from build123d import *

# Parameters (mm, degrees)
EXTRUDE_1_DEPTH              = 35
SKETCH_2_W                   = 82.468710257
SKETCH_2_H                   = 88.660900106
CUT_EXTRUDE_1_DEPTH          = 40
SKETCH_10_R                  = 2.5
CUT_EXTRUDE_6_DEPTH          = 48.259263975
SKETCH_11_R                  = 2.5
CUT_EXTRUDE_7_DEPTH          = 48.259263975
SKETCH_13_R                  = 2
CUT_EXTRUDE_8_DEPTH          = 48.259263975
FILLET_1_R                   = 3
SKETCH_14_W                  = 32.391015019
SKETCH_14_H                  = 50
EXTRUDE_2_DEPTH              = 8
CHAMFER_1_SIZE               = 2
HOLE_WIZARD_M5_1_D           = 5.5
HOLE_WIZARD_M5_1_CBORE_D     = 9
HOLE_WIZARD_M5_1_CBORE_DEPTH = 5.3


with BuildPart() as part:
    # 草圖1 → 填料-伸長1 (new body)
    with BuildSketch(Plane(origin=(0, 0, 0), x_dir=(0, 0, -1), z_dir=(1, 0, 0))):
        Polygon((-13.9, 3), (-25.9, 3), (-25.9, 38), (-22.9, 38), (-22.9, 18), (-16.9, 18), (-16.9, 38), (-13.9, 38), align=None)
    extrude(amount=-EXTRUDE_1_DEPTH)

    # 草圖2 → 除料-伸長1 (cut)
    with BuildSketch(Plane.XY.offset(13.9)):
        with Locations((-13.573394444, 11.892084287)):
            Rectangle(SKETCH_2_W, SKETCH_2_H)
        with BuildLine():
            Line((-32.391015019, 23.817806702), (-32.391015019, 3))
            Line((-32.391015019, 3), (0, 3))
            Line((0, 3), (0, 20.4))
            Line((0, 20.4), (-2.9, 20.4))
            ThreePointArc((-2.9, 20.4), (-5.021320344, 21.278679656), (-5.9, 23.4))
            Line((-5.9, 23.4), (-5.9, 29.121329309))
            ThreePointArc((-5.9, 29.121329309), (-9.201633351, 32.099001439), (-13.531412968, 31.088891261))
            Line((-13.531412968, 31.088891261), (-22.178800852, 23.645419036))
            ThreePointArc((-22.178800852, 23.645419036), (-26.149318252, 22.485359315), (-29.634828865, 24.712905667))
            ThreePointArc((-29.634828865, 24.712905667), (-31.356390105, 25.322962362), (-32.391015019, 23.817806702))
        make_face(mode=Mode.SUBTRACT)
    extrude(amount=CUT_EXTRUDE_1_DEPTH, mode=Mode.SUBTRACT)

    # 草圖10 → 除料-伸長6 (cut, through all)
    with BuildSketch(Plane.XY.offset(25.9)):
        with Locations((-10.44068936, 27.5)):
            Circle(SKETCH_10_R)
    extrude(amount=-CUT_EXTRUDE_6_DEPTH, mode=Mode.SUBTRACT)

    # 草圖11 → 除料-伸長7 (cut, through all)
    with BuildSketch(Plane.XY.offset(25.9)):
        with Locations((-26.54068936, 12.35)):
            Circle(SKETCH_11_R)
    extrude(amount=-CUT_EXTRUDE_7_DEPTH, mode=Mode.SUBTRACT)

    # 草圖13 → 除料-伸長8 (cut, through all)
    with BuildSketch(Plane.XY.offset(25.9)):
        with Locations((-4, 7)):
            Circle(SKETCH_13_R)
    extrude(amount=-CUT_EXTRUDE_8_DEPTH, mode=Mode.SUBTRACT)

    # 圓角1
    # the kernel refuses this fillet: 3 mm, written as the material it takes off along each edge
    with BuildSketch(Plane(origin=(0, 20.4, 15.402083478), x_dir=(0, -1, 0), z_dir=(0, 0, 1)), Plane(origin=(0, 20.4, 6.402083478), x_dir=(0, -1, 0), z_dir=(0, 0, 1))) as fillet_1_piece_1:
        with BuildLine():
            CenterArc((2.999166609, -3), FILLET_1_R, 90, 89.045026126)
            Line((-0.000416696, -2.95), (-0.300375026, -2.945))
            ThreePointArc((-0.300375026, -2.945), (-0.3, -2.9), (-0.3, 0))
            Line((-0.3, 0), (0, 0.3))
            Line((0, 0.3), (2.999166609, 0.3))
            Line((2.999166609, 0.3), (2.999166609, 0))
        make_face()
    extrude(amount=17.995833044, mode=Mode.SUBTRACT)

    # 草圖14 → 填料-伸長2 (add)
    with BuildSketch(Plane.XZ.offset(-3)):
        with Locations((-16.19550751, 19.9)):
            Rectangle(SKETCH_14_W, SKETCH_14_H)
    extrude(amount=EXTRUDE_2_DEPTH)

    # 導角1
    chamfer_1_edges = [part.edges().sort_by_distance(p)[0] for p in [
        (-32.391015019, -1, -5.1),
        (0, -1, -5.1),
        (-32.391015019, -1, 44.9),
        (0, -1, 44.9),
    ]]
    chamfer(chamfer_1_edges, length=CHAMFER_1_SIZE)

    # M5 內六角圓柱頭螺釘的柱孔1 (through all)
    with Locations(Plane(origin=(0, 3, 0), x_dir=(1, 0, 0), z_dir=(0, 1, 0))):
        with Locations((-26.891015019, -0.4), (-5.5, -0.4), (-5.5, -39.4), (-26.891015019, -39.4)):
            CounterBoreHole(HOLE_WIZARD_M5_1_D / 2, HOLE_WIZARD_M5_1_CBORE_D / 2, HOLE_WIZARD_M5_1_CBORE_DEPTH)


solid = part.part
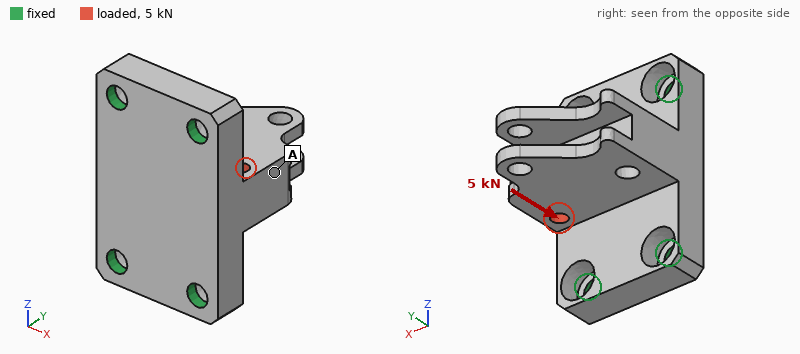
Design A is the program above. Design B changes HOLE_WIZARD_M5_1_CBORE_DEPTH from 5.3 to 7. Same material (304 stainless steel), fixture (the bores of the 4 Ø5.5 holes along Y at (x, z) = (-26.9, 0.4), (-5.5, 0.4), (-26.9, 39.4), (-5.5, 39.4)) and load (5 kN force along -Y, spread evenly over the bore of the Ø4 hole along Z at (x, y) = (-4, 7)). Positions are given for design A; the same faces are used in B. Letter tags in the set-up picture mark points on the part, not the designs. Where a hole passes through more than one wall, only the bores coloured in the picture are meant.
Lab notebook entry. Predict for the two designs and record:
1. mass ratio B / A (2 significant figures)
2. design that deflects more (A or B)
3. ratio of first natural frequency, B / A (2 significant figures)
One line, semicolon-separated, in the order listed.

0.99; B; 0.75
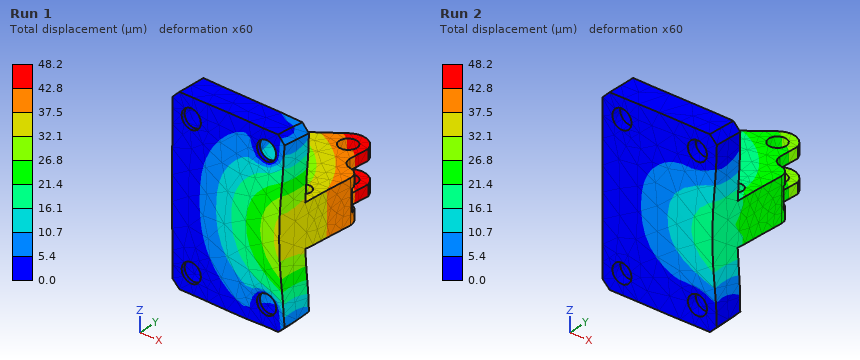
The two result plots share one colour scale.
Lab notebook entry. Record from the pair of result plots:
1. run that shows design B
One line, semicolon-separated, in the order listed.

Run 1
